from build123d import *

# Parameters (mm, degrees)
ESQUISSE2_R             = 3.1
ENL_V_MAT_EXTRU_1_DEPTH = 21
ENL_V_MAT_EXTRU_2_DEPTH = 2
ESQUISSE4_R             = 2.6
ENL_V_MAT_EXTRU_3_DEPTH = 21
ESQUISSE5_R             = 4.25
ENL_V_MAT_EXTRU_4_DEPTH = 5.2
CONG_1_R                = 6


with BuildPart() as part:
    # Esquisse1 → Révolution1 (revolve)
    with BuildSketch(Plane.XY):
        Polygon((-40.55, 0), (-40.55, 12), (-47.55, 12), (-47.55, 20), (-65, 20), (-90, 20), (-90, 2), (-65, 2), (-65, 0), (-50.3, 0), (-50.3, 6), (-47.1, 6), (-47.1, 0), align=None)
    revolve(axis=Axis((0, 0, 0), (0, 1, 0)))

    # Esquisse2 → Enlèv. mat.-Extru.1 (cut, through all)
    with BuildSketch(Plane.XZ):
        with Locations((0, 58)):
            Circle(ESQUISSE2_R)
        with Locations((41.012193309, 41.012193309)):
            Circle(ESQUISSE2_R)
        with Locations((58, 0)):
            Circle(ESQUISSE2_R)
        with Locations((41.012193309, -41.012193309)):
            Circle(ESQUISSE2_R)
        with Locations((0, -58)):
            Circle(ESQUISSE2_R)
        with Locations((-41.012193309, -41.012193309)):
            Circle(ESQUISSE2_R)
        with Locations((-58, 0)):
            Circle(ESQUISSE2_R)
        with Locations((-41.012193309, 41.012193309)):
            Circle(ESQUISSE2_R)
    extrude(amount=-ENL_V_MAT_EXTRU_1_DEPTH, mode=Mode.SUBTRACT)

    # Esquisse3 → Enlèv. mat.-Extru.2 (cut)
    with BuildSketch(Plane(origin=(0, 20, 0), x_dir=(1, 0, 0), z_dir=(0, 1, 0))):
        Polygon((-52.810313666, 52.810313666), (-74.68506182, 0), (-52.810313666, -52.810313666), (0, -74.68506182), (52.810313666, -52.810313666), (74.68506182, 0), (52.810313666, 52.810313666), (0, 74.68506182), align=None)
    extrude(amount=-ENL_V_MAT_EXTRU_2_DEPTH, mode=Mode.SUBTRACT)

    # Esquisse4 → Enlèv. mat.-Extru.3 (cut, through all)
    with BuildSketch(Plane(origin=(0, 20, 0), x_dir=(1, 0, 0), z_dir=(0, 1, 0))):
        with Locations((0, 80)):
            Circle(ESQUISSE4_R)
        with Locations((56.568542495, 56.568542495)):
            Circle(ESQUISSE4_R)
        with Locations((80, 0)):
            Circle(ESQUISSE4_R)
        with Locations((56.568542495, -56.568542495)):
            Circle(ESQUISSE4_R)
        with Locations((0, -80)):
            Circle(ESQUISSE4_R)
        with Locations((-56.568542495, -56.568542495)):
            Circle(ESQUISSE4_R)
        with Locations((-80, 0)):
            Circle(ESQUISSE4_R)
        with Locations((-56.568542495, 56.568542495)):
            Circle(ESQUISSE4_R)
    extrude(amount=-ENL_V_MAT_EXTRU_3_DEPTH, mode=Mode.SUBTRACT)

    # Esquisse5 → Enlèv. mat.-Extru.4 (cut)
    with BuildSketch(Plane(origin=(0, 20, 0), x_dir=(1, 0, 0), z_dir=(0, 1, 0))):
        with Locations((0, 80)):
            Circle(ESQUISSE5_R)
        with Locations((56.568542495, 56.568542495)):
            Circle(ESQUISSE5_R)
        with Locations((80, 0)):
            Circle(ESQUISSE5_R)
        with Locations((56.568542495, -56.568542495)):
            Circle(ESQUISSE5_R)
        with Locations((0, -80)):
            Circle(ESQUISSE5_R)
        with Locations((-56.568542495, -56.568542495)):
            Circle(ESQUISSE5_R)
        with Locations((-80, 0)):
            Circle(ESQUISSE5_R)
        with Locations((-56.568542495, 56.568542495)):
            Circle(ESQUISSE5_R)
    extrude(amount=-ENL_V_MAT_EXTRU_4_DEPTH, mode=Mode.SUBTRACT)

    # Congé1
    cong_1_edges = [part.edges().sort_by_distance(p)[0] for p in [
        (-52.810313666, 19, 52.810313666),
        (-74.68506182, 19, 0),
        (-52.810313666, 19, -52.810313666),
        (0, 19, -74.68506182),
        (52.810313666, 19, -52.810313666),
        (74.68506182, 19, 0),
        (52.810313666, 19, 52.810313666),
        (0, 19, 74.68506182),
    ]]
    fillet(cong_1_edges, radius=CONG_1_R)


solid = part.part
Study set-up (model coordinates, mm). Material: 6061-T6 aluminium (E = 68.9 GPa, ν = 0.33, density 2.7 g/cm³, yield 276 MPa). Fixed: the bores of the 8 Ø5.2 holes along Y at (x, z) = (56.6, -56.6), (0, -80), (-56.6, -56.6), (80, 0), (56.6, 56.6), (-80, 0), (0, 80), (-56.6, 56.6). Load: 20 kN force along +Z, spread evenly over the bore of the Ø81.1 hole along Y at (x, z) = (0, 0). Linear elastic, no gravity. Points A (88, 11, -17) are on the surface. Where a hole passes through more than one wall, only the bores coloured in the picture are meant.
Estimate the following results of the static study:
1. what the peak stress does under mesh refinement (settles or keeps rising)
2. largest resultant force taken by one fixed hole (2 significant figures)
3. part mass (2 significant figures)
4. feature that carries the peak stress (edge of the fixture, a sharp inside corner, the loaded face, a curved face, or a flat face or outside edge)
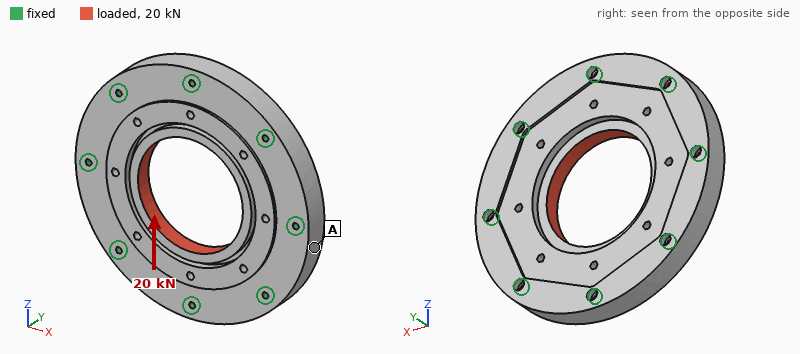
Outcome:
keeps rising
3.5 kN
900 g
edge of the fixture
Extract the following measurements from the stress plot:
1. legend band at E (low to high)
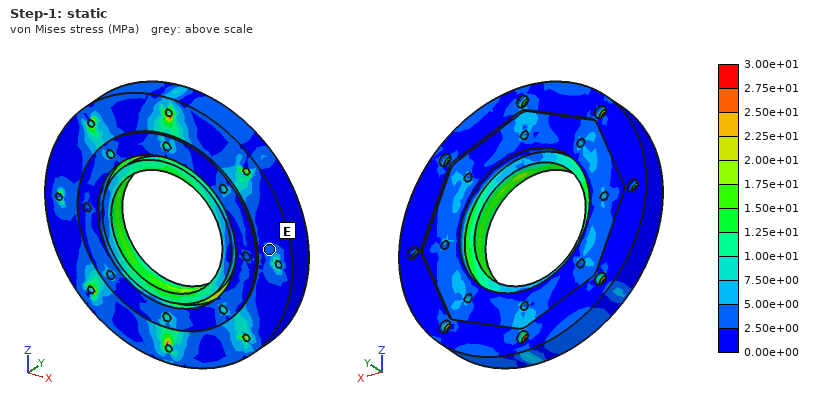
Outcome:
2.50e+00 to 5.00e+00 MPa
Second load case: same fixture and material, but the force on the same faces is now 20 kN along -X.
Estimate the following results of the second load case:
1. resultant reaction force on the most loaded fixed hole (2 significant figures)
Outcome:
3.5 kN
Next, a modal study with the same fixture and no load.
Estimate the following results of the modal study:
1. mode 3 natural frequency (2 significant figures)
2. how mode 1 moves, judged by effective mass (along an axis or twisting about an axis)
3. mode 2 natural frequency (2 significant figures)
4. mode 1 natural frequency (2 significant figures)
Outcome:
7800 Hz
along Y
7800 Hz
6100 Hz
